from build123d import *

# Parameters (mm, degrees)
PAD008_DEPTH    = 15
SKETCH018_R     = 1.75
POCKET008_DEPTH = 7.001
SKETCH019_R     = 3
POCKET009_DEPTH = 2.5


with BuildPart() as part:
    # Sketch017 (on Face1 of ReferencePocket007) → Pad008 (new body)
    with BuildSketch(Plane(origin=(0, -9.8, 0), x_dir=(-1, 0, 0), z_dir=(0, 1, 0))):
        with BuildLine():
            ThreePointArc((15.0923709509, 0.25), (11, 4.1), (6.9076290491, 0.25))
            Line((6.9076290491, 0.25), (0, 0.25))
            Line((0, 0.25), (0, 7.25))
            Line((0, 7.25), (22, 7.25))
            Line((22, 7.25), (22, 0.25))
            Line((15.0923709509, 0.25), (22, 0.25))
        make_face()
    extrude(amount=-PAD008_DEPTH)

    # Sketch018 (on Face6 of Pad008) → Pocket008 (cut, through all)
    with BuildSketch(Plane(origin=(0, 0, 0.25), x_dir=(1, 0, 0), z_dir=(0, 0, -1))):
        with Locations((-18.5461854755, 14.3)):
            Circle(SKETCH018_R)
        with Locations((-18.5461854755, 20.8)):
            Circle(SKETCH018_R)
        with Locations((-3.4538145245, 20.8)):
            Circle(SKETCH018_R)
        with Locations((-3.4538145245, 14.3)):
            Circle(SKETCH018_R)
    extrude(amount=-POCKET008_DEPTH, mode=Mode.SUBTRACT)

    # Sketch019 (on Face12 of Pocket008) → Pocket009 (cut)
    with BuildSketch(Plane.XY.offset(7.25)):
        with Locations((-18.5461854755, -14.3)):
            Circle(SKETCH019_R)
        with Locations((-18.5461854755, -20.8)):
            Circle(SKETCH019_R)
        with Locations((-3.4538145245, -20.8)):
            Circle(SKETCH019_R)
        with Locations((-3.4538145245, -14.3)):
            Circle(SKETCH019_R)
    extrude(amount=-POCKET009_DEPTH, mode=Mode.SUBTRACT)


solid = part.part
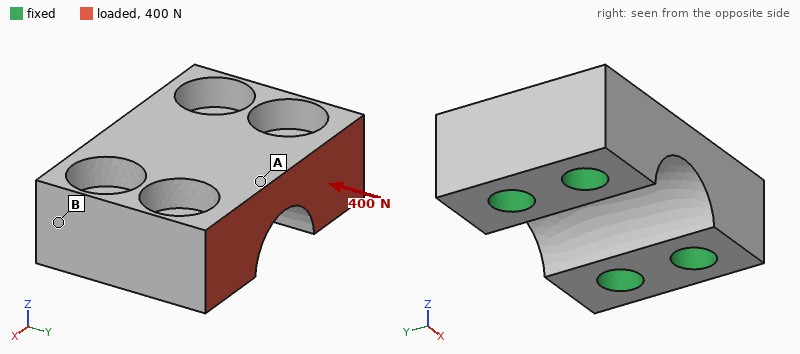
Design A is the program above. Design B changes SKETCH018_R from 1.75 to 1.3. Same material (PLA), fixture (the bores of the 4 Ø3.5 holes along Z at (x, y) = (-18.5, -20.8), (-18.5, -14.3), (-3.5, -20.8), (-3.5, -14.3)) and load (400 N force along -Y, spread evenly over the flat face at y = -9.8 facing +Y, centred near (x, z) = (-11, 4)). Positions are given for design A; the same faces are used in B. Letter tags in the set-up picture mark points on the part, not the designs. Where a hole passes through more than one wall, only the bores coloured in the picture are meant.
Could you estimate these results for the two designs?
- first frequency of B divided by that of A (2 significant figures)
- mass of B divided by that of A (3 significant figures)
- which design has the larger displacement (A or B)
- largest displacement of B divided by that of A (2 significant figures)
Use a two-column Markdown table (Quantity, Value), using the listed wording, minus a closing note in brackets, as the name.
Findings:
| Quantity | Value |
|---|---|
| first frequency of B divided by that of A | 0.88 |
| mass of B divided by that of A | 1.05 |
| which design has the larger displacement | B |
| largest displacement of B divided by that of A | 1.1 |
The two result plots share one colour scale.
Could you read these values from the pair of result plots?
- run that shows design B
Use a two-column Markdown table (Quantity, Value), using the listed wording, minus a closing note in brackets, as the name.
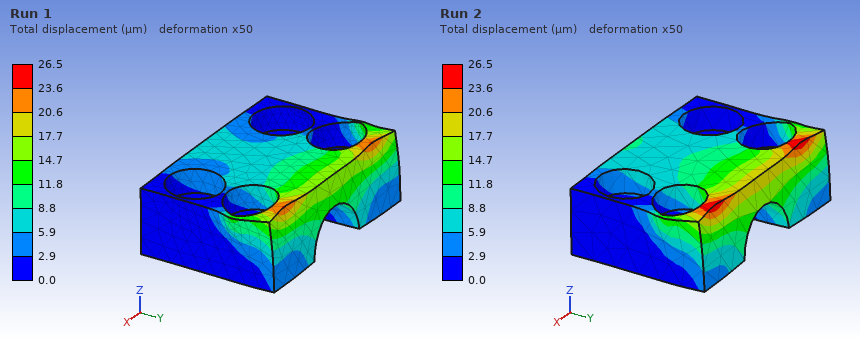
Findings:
| Quantity | Value |
|---|---|
| run that shows design B | Run 2 |
